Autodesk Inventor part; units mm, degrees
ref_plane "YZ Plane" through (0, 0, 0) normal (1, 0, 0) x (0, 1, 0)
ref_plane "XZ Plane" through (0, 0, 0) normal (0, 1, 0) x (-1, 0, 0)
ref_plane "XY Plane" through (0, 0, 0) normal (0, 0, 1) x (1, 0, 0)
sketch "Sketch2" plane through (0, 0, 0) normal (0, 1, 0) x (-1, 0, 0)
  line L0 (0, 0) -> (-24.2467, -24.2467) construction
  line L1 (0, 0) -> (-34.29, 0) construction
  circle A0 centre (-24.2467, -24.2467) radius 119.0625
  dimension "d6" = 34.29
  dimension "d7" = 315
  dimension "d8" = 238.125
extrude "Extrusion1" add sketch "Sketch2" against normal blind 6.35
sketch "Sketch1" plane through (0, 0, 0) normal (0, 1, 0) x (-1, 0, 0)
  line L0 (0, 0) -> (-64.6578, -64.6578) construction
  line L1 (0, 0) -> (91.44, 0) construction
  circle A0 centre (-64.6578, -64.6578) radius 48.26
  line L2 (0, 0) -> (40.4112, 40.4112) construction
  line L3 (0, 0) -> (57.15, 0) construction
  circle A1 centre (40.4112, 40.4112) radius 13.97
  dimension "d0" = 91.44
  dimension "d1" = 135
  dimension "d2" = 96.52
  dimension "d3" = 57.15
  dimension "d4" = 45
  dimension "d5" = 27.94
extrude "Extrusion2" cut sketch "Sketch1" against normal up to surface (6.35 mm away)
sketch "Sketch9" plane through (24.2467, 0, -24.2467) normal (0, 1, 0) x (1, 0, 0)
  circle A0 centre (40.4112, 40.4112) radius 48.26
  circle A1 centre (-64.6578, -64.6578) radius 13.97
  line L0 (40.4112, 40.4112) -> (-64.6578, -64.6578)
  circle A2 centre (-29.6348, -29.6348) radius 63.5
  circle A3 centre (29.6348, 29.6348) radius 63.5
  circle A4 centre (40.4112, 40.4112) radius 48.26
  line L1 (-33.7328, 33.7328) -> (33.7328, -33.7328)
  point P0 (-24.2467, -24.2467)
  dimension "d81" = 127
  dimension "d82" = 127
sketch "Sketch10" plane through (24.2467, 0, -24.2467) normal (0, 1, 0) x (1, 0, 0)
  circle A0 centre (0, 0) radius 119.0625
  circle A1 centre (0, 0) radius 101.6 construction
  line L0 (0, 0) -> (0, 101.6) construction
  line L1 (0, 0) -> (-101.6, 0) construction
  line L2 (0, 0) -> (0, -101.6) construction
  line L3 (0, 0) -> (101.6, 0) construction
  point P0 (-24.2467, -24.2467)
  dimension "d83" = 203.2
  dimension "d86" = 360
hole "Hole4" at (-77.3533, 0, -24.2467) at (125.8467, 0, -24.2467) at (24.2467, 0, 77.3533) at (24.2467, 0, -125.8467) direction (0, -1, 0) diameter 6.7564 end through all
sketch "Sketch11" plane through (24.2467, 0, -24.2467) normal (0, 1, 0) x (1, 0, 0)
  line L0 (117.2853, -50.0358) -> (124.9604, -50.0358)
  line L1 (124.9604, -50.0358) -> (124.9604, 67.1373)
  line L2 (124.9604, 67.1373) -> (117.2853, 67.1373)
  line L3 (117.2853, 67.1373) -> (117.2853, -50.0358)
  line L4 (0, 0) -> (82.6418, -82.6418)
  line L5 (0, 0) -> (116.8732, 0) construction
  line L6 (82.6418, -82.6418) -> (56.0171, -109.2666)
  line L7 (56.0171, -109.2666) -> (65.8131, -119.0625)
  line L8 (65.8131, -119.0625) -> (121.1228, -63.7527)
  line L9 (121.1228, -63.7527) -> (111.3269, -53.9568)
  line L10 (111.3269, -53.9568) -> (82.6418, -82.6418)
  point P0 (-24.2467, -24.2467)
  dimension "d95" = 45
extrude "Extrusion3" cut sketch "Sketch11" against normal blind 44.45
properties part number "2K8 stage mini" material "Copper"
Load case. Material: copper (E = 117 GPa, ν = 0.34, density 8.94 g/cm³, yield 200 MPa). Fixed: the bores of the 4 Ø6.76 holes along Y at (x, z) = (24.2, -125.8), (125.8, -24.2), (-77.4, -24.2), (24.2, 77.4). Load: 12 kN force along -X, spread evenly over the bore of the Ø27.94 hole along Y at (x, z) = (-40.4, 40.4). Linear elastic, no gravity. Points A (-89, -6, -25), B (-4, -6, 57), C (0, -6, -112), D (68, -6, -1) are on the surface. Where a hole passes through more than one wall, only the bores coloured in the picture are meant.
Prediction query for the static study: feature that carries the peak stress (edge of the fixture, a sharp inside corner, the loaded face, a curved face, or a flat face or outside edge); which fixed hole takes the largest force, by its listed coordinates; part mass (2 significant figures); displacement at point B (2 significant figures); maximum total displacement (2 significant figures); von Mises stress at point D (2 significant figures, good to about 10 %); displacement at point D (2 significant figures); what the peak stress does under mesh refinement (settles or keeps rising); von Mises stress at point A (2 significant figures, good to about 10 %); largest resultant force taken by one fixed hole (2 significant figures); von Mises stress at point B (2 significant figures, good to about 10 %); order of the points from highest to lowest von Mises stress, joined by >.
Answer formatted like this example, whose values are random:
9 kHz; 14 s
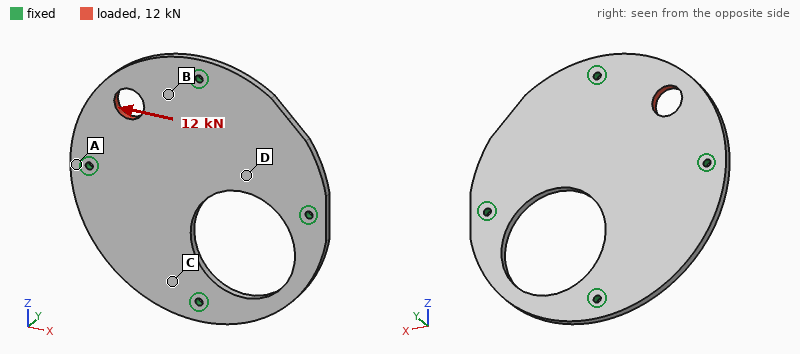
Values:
edge of the fixture; (24.2, 77.4); 2.1 kg; 9.9 µm; 25 µm; 8.2 MPa; 5.6 µm; keeps rising; 15 MPa; 6.1 kN; 23 MPa; B > A > D > C
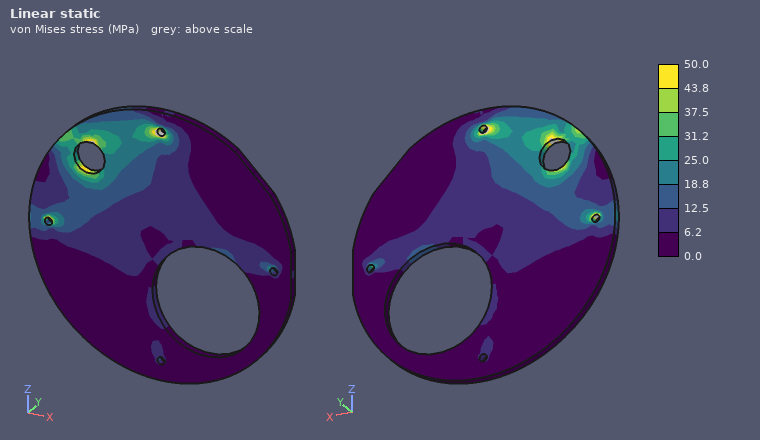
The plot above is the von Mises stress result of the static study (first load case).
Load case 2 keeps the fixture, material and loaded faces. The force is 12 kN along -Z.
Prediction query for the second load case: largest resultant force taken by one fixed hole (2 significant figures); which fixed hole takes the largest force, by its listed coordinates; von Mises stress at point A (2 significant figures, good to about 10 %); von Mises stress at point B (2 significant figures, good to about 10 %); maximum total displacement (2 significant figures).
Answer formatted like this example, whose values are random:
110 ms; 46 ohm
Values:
6.1 kN; (-77.4, -24.2); 6.2 MPa; 13 MPa; 25 µm
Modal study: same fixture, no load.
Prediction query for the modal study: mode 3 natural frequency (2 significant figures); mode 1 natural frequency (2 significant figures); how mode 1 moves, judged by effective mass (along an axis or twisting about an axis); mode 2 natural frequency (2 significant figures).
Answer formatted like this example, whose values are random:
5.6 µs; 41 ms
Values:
900 Hz; 770 Hz; along Y; 860 Hz
